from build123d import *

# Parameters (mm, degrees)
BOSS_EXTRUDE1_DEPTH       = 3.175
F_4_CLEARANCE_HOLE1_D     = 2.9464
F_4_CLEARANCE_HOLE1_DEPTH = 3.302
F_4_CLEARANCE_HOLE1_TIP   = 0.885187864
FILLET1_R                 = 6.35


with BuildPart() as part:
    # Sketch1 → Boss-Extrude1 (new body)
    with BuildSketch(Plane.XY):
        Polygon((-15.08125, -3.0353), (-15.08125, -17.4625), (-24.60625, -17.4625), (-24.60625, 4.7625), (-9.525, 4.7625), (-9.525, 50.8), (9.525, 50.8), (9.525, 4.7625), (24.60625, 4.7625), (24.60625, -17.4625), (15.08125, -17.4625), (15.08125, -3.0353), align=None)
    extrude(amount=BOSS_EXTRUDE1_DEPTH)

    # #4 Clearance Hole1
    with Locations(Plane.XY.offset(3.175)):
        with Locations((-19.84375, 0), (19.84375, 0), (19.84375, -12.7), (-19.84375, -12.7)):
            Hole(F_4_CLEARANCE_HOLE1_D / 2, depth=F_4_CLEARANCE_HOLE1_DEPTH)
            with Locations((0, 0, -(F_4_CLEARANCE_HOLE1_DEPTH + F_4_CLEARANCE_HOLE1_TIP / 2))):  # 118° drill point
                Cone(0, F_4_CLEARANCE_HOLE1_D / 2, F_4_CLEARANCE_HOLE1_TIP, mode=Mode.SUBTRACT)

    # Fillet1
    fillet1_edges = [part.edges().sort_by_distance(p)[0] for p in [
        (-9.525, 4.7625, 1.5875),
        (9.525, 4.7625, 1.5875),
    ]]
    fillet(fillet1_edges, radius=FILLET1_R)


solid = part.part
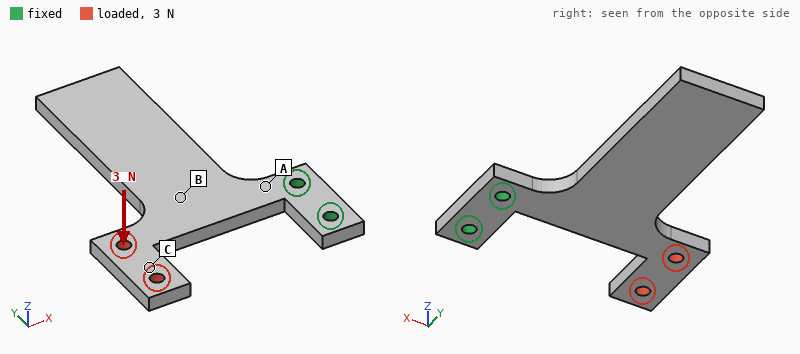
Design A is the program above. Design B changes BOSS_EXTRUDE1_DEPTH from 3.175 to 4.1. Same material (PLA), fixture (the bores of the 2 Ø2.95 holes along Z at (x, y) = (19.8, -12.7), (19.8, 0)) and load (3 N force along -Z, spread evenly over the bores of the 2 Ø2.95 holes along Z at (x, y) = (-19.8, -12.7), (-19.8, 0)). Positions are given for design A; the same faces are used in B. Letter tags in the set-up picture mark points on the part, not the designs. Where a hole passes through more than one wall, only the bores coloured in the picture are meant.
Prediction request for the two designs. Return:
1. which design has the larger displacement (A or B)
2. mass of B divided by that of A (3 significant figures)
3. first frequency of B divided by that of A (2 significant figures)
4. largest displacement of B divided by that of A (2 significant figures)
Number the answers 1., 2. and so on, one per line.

1. A
2. 1.29
3. 1.3
4. 0.48
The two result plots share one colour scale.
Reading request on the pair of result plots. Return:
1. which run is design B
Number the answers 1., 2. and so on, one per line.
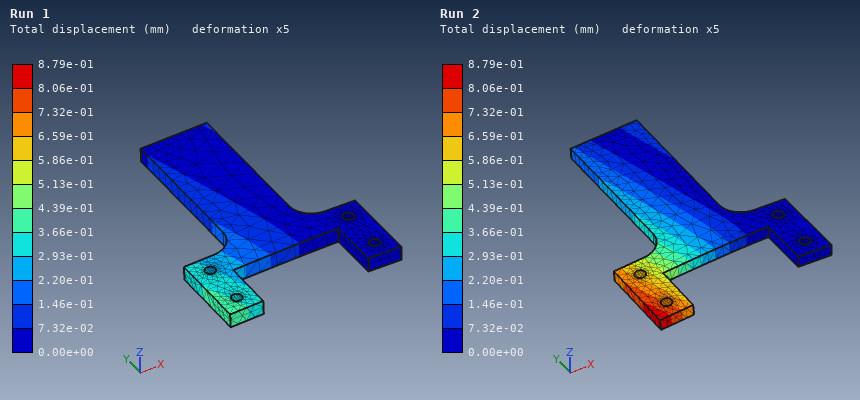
1. Run 1
